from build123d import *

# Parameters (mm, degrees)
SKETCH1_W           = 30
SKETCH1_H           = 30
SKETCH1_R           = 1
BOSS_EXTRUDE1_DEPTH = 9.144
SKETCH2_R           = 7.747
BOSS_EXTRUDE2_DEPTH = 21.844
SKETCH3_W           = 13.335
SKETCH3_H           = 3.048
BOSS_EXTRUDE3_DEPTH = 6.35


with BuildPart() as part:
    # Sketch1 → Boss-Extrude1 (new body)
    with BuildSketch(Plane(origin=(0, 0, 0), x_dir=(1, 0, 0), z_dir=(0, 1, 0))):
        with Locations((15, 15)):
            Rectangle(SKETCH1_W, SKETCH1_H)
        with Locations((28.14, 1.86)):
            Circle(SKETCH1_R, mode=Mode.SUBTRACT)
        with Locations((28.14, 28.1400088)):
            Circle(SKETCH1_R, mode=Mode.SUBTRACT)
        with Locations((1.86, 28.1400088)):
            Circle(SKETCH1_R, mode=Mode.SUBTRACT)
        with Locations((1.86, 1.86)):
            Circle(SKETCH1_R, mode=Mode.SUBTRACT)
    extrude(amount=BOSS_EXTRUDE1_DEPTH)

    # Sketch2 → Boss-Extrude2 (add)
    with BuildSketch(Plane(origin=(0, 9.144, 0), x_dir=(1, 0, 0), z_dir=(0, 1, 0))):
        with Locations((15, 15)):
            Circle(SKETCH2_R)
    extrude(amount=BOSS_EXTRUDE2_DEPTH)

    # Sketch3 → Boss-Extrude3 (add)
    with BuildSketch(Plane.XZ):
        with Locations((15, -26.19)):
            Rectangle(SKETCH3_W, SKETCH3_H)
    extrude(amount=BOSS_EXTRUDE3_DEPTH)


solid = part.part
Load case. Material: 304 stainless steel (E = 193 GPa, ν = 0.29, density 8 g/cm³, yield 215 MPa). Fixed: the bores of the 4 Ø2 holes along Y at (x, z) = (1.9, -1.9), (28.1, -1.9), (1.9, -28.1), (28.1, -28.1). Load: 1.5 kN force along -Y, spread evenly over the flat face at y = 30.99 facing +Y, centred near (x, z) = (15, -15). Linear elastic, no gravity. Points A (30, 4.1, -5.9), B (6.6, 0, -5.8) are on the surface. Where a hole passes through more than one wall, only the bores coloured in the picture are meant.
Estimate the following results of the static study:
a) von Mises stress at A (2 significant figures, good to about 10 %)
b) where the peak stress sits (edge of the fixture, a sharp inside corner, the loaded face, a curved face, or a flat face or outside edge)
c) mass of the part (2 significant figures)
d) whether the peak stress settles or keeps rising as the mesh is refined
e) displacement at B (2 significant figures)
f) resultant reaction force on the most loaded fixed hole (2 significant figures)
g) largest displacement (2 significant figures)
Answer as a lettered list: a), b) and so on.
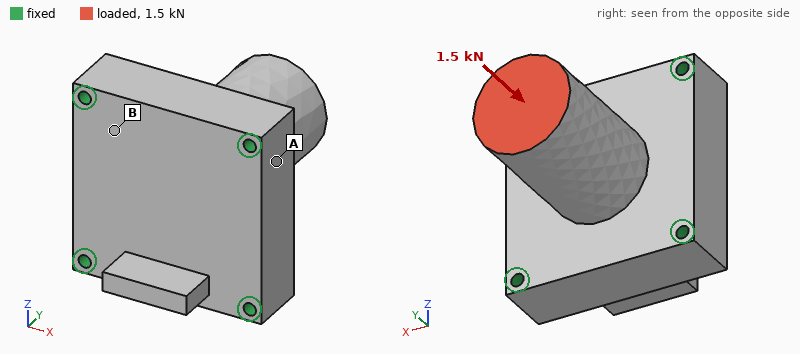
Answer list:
a) 7.8 MPa
b) edge of the fixture
c) 100 g
d) keeps rising
e) 0.77 µm
f) 380 N
g) 2.3 µm
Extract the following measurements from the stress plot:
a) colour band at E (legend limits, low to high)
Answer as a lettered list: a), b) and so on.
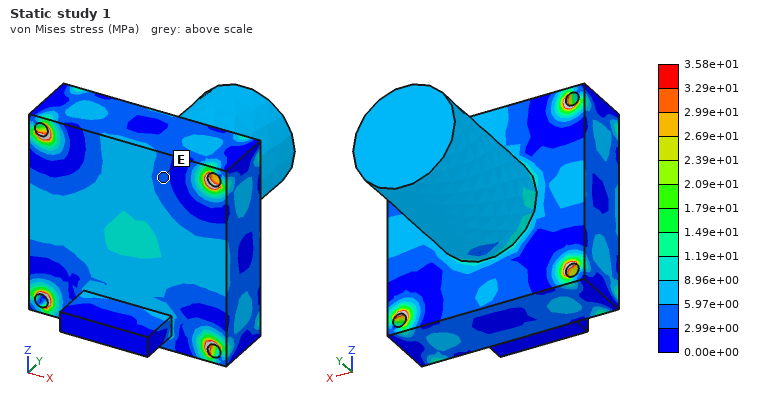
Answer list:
a) 2.99e+00 to 5.97e+00 MPa
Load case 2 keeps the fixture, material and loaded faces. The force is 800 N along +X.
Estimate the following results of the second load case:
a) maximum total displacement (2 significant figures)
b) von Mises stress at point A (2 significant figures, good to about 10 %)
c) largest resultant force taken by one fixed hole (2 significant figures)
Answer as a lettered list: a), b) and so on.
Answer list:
a) 13 µm
b) 18 MPa
c) 490 N
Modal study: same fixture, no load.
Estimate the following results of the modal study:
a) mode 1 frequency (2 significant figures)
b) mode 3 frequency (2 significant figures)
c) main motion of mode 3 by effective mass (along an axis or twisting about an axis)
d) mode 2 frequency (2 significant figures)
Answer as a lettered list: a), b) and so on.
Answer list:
a) 12 kHz
b) 20 kHz
c) along Y
d) 12 kHz
